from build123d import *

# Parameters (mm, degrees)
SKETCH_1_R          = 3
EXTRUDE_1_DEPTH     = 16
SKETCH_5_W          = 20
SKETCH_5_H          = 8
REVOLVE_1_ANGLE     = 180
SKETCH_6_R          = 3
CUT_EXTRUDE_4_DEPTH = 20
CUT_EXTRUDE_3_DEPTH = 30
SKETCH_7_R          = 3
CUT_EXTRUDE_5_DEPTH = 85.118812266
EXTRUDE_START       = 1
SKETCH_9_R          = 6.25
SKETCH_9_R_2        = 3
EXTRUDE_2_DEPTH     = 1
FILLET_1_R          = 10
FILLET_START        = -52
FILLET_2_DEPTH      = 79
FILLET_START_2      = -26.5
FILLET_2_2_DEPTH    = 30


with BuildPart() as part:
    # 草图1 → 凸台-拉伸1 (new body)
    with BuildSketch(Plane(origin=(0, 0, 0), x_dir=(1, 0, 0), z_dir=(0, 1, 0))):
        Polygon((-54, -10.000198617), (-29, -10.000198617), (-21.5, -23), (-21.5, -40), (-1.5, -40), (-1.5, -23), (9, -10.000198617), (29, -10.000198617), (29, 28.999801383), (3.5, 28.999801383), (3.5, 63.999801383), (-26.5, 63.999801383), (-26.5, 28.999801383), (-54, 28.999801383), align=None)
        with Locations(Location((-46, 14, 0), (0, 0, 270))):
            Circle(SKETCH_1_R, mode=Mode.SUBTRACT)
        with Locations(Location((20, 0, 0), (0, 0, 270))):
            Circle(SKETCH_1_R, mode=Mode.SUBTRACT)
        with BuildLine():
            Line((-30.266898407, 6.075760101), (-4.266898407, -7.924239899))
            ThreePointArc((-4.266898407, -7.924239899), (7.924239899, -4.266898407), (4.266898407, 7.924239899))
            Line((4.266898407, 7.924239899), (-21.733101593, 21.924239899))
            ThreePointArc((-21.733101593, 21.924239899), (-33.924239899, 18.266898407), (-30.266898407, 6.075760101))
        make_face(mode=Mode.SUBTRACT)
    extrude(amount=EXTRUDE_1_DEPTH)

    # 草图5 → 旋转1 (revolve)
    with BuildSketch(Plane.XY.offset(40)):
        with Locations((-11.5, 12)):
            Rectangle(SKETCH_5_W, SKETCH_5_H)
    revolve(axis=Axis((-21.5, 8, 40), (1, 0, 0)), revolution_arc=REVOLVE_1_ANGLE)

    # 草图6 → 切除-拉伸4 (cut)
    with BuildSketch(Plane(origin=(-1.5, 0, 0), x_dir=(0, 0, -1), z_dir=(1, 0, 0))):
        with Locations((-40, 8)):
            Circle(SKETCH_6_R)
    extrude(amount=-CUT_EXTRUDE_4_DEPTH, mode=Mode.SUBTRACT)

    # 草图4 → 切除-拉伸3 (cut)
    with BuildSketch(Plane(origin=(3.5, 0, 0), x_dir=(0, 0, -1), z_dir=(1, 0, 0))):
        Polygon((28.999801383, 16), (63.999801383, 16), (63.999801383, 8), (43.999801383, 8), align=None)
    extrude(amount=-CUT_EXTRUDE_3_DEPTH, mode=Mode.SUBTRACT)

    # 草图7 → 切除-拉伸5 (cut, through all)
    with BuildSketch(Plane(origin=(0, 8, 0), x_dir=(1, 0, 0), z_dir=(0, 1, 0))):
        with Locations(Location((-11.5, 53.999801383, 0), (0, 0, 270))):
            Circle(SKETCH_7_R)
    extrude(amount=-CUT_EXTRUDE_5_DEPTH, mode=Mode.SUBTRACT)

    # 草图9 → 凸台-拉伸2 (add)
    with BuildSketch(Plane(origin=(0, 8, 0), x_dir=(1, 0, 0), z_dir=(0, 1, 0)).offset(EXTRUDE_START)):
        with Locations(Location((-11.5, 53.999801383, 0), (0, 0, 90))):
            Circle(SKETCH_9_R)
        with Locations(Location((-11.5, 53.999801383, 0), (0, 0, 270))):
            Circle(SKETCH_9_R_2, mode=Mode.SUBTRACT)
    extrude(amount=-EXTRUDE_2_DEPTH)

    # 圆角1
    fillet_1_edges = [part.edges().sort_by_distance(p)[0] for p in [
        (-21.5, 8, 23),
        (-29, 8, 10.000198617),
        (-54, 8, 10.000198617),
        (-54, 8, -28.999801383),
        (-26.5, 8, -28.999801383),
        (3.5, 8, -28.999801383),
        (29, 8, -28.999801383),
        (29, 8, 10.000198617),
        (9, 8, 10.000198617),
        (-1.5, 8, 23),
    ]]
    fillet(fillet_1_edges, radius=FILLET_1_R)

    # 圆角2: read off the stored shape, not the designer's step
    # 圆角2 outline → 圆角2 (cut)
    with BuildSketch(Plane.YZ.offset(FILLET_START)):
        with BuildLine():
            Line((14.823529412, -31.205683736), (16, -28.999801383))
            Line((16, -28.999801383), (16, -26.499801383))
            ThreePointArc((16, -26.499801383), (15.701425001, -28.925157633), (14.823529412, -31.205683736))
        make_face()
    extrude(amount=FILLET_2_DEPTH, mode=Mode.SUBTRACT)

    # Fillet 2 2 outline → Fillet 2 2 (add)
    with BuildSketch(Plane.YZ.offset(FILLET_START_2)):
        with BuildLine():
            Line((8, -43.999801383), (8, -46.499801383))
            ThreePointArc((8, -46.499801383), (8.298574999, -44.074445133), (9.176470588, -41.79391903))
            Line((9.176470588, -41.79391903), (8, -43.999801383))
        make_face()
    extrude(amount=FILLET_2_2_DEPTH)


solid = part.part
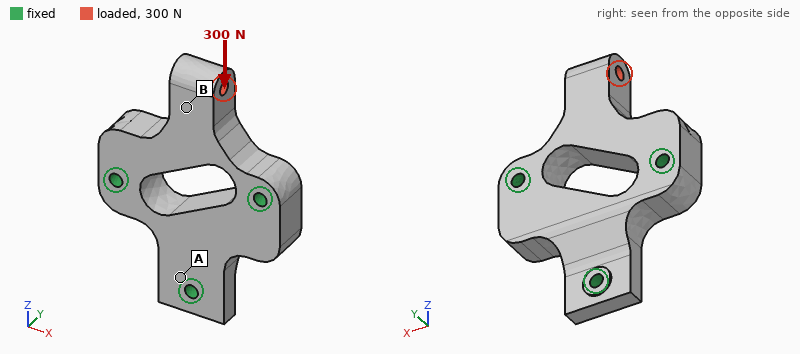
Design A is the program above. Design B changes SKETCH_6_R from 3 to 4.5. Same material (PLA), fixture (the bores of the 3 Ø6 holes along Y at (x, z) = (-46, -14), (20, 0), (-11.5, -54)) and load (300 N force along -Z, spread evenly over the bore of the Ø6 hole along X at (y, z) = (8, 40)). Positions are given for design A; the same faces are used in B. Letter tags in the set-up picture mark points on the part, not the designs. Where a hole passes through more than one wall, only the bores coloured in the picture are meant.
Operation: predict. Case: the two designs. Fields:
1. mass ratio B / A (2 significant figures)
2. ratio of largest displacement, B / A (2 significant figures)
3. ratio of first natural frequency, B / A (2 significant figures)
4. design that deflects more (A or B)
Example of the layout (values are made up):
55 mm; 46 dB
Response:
0.99; 1.1; 1.1; B
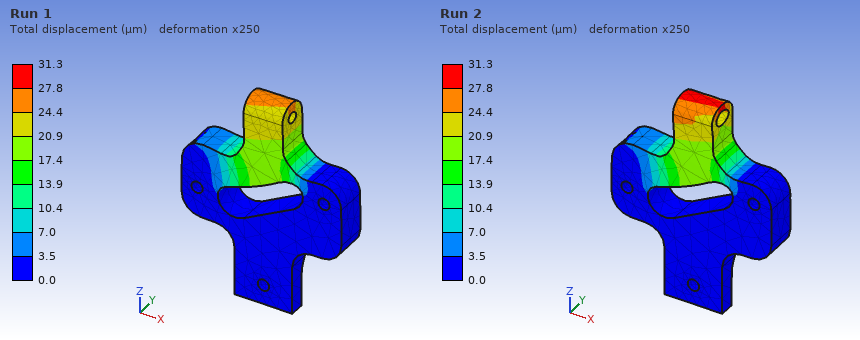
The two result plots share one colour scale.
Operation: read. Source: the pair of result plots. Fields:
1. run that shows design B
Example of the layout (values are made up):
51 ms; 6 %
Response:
Run 2
